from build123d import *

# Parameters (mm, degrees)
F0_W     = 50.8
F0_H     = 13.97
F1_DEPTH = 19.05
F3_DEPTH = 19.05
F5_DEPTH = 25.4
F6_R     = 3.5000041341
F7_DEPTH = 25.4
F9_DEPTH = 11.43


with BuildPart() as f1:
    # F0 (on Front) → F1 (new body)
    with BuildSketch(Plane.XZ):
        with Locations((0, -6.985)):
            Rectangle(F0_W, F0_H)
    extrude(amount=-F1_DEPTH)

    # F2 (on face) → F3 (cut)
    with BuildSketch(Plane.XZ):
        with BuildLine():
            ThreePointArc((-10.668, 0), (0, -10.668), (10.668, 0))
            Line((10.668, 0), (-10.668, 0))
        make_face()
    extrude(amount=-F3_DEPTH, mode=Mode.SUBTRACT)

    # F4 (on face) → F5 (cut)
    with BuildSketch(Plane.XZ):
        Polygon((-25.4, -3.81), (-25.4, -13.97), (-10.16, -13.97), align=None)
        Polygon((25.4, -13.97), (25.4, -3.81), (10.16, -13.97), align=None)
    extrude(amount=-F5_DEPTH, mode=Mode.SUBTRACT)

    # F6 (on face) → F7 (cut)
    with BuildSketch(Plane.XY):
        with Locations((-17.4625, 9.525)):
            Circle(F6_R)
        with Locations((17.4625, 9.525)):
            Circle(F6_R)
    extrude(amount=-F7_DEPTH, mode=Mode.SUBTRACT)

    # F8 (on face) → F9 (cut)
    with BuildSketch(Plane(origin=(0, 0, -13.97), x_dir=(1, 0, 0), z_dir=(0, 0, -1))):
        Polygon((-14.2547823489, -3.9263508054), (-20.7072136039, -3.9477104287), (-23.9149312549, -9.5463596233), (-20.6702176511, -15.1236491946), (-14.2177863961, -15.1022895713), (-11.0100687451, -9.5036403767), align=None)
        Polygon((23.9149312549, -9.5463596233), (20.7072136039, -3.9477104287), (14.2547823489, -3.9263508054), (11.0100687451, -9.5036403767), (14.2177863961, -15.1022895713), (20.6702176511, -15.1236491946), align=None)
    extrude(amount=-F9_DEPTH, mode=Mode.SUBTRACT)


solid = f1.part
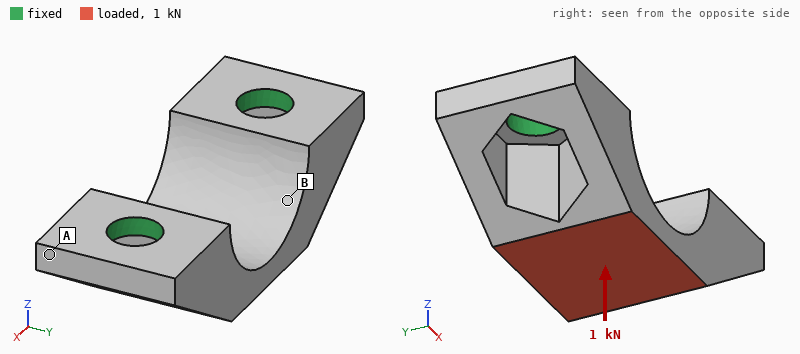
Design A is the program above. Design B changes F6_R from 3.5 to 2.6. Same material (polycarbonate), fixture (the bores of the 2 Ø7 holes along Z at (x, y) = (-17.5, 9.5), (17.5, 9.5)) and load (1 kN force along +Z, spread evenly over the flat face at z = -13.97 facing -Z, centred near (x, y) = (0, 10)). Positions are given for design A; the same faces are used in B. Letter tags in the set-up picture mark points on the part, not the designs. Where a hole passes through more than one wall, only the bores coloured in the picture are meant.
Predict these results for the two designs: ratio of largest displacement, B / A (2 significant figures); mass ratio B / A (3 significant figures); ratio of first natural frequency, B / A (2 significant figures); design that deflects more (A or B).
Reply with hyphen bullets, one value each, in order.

- 1.3
- 1.02
- 0.77
- B
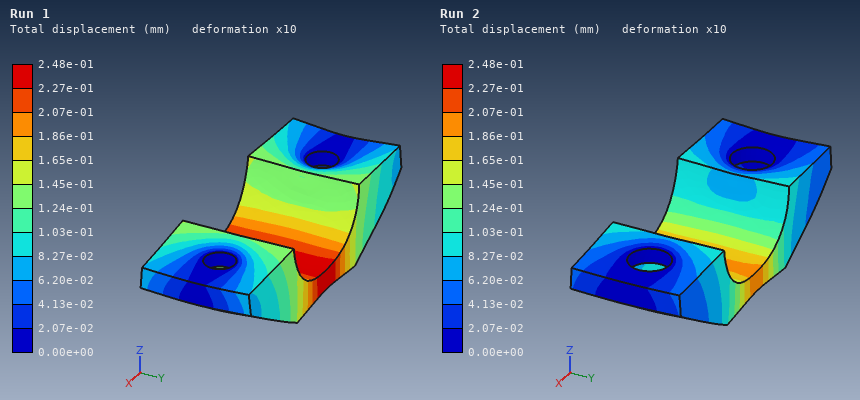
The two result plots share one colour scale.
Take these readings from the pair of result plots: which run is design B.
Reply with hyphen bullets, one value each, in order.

- Run 1
